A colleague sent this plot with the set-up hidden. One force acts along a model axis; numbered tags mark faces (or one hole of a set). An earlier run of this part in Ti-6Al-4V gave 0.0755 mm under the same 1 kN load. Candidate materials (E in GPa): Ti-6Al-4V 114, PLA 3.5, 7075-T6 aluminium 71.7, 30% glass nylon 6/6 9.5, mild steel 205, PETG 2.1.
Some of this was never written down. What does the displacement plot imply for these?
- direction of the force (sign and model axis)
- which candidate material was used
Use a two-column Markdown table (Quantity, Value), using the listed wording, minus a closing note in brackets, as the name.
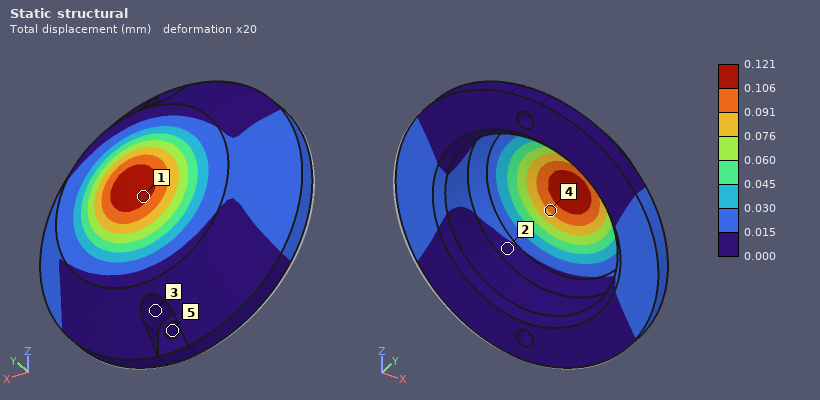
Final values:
| Quantity | Value |
|---|---|
| direction of the force | +Y |
| which candidate material was used | 7075-T6 aluminium |
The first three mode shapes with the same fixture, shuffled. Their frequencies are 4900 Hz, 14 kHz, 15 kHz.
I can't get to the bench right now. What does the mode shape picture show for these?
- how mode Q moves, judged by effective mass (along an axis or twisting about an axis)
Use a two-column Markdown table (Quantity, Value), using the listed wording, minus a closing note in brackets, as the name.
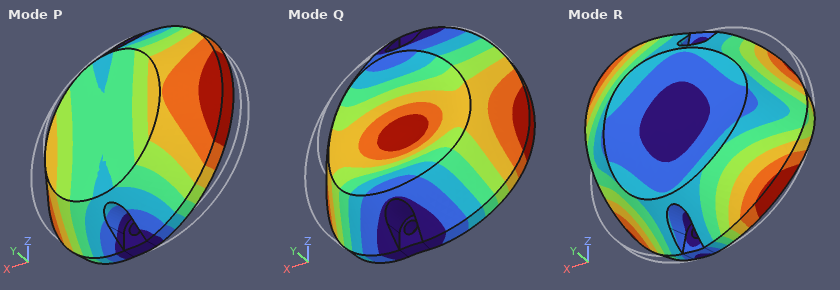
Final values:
| Quantity | Value |
|---|---|
| how mode Q moves, judged by effective mass | along Y |
